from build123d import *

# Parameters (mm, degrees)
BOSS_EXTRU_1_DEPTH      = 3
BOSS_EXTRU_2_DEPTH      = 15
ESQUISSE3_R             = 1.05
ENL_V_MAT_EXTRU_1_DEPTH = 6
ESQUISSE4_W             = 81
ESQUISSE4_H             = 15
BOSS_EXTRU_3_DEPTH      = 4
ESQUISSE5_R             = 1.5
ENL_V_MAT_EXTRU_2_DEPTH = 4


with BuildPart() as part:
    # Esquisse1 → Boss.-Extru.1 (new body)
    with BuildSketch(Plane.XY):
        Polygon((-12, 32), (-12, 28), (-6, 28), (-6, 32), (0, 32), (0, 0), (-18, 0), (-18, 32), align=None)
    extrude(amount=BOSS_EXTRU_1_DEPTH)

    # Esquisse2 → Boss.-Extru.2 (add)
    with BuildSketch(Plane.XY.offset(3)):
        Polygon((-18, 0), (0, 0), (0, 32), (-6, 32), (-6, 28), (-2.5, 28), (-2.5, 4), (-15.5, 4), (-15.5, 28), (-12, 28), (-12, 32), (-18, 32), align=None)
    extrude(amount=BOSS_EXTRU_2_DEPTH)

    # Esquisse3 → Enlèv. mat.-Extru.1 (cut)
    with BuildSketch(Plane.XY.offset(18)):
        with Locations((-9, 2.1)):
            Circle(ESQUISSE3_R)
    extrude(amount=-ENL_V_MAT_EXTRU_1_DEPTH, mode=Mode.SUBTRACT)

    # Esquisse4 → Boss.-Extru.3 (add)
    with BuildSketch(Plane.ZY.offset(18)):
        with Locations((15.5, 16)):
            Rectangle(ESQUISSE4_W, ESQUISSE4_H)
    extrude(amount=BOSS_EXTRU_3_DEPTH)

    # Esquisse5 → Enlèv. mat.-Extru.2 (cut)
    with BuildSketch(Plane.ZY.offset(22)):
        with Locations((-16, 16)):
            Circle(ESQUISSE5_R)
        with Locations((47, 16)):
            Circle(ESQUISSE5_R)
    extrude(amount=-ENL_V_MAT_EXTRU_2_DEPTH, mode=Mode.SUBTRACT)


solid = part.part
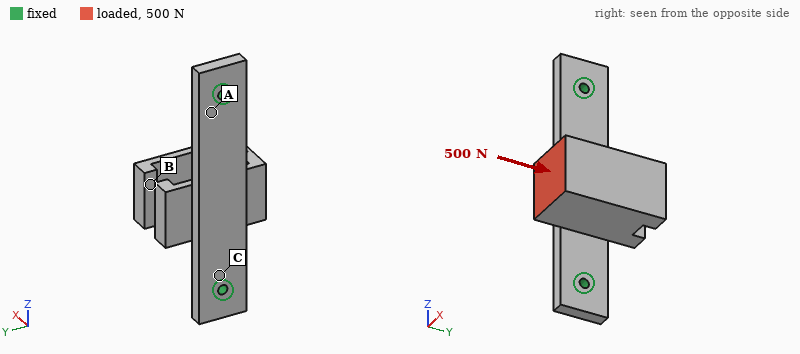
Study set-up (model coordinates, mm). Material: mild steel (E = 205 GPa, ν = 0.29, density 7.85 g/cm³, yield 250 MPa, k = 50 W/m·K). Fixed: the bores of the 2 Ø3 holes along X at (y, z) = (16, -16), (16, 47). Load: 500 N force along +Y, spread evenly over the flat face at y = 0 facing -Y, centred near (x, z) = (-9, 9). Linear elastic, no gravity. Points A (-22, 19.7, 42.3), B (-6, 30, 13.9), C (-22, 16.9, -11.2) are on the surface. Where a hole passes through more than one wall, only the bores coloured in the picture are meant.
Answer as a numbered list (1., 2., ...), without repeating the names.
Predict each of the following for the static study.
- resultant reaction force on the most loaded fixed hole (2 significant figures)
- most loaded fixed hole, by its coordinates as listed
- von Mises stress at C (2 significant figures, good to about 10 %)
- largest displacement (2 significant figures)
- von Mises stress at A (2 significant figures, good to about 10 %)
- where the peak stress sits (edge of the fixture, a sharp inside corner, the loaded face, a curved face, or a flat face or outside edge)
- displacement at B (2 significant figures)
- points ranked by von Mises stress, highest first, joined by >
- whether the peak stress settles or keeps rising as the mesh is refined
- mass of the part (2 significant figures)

1. 310 N
2. (16, -16)
3. 66 MPa
4. 78 µm
5. 31 MPa
6. edge of the fixture
7. 59 µm
8. C > A > B
9. keeps rising
10. 79 g
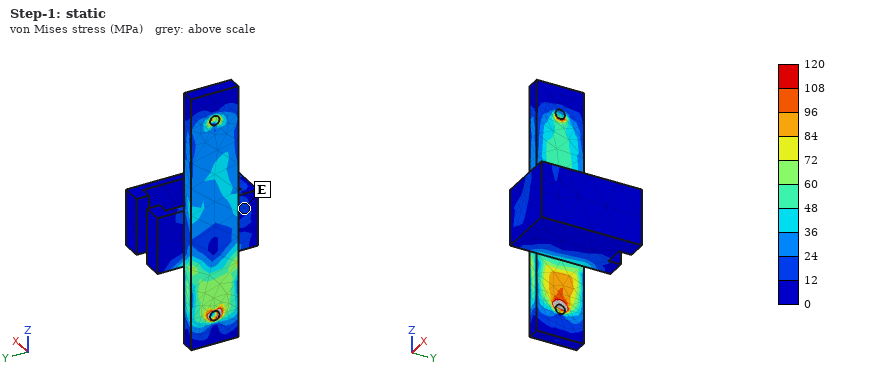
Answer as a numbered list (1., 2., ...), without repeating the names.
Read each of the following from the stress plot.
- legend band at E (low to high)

1. 12 to 24 MPa
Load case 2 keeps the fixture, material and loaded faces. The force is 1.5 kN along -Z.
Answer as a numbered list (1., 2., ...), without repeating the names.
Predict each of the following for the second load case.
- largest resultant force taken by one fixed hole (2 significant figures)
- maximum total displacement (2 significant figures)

1. 960 N
2. 91 µm
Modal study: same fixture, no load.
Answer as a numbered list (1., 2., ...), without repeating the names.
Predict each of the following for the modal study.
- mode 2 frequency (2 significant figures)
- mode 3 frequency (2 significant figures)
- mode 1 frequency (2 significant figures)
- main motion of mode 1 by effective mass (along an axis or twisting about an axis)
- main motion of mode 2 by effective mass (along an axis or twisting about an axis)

1. 2800 Hz
2. 4900 Hz
3. 2100 Hz
4. along Y
5. along X
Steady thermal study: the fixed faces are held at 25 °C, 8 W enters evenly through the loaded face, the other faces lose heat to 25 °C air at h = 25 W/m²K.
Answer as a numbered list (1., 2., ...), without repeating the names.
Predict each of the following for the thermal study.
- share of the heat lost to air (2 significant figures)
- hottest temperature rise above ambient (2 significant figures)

1. 38 %
2. 41 K
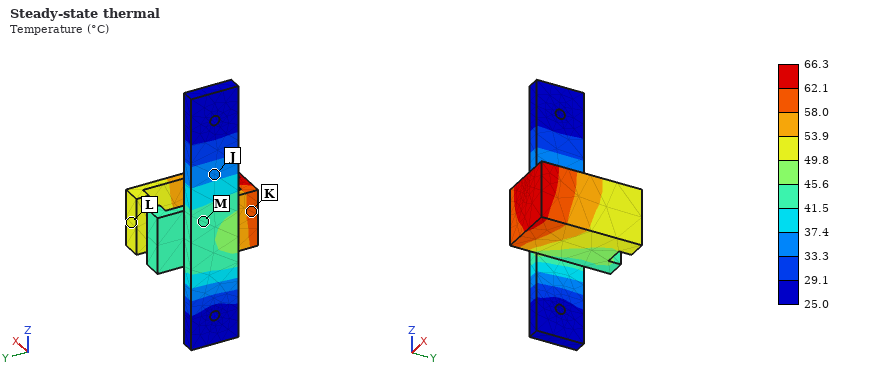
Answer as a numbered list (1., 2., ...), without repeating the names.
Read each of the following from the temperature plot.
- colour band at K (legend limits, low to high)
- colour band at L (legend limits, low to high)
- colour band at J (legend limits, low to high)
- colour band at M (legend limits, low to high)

1. 58.0 to 62.1 °C
2. 49.8 to 53.9 °C
3. 33.3 to 37.4 °C
4. 41.5 to 45.6 °C
